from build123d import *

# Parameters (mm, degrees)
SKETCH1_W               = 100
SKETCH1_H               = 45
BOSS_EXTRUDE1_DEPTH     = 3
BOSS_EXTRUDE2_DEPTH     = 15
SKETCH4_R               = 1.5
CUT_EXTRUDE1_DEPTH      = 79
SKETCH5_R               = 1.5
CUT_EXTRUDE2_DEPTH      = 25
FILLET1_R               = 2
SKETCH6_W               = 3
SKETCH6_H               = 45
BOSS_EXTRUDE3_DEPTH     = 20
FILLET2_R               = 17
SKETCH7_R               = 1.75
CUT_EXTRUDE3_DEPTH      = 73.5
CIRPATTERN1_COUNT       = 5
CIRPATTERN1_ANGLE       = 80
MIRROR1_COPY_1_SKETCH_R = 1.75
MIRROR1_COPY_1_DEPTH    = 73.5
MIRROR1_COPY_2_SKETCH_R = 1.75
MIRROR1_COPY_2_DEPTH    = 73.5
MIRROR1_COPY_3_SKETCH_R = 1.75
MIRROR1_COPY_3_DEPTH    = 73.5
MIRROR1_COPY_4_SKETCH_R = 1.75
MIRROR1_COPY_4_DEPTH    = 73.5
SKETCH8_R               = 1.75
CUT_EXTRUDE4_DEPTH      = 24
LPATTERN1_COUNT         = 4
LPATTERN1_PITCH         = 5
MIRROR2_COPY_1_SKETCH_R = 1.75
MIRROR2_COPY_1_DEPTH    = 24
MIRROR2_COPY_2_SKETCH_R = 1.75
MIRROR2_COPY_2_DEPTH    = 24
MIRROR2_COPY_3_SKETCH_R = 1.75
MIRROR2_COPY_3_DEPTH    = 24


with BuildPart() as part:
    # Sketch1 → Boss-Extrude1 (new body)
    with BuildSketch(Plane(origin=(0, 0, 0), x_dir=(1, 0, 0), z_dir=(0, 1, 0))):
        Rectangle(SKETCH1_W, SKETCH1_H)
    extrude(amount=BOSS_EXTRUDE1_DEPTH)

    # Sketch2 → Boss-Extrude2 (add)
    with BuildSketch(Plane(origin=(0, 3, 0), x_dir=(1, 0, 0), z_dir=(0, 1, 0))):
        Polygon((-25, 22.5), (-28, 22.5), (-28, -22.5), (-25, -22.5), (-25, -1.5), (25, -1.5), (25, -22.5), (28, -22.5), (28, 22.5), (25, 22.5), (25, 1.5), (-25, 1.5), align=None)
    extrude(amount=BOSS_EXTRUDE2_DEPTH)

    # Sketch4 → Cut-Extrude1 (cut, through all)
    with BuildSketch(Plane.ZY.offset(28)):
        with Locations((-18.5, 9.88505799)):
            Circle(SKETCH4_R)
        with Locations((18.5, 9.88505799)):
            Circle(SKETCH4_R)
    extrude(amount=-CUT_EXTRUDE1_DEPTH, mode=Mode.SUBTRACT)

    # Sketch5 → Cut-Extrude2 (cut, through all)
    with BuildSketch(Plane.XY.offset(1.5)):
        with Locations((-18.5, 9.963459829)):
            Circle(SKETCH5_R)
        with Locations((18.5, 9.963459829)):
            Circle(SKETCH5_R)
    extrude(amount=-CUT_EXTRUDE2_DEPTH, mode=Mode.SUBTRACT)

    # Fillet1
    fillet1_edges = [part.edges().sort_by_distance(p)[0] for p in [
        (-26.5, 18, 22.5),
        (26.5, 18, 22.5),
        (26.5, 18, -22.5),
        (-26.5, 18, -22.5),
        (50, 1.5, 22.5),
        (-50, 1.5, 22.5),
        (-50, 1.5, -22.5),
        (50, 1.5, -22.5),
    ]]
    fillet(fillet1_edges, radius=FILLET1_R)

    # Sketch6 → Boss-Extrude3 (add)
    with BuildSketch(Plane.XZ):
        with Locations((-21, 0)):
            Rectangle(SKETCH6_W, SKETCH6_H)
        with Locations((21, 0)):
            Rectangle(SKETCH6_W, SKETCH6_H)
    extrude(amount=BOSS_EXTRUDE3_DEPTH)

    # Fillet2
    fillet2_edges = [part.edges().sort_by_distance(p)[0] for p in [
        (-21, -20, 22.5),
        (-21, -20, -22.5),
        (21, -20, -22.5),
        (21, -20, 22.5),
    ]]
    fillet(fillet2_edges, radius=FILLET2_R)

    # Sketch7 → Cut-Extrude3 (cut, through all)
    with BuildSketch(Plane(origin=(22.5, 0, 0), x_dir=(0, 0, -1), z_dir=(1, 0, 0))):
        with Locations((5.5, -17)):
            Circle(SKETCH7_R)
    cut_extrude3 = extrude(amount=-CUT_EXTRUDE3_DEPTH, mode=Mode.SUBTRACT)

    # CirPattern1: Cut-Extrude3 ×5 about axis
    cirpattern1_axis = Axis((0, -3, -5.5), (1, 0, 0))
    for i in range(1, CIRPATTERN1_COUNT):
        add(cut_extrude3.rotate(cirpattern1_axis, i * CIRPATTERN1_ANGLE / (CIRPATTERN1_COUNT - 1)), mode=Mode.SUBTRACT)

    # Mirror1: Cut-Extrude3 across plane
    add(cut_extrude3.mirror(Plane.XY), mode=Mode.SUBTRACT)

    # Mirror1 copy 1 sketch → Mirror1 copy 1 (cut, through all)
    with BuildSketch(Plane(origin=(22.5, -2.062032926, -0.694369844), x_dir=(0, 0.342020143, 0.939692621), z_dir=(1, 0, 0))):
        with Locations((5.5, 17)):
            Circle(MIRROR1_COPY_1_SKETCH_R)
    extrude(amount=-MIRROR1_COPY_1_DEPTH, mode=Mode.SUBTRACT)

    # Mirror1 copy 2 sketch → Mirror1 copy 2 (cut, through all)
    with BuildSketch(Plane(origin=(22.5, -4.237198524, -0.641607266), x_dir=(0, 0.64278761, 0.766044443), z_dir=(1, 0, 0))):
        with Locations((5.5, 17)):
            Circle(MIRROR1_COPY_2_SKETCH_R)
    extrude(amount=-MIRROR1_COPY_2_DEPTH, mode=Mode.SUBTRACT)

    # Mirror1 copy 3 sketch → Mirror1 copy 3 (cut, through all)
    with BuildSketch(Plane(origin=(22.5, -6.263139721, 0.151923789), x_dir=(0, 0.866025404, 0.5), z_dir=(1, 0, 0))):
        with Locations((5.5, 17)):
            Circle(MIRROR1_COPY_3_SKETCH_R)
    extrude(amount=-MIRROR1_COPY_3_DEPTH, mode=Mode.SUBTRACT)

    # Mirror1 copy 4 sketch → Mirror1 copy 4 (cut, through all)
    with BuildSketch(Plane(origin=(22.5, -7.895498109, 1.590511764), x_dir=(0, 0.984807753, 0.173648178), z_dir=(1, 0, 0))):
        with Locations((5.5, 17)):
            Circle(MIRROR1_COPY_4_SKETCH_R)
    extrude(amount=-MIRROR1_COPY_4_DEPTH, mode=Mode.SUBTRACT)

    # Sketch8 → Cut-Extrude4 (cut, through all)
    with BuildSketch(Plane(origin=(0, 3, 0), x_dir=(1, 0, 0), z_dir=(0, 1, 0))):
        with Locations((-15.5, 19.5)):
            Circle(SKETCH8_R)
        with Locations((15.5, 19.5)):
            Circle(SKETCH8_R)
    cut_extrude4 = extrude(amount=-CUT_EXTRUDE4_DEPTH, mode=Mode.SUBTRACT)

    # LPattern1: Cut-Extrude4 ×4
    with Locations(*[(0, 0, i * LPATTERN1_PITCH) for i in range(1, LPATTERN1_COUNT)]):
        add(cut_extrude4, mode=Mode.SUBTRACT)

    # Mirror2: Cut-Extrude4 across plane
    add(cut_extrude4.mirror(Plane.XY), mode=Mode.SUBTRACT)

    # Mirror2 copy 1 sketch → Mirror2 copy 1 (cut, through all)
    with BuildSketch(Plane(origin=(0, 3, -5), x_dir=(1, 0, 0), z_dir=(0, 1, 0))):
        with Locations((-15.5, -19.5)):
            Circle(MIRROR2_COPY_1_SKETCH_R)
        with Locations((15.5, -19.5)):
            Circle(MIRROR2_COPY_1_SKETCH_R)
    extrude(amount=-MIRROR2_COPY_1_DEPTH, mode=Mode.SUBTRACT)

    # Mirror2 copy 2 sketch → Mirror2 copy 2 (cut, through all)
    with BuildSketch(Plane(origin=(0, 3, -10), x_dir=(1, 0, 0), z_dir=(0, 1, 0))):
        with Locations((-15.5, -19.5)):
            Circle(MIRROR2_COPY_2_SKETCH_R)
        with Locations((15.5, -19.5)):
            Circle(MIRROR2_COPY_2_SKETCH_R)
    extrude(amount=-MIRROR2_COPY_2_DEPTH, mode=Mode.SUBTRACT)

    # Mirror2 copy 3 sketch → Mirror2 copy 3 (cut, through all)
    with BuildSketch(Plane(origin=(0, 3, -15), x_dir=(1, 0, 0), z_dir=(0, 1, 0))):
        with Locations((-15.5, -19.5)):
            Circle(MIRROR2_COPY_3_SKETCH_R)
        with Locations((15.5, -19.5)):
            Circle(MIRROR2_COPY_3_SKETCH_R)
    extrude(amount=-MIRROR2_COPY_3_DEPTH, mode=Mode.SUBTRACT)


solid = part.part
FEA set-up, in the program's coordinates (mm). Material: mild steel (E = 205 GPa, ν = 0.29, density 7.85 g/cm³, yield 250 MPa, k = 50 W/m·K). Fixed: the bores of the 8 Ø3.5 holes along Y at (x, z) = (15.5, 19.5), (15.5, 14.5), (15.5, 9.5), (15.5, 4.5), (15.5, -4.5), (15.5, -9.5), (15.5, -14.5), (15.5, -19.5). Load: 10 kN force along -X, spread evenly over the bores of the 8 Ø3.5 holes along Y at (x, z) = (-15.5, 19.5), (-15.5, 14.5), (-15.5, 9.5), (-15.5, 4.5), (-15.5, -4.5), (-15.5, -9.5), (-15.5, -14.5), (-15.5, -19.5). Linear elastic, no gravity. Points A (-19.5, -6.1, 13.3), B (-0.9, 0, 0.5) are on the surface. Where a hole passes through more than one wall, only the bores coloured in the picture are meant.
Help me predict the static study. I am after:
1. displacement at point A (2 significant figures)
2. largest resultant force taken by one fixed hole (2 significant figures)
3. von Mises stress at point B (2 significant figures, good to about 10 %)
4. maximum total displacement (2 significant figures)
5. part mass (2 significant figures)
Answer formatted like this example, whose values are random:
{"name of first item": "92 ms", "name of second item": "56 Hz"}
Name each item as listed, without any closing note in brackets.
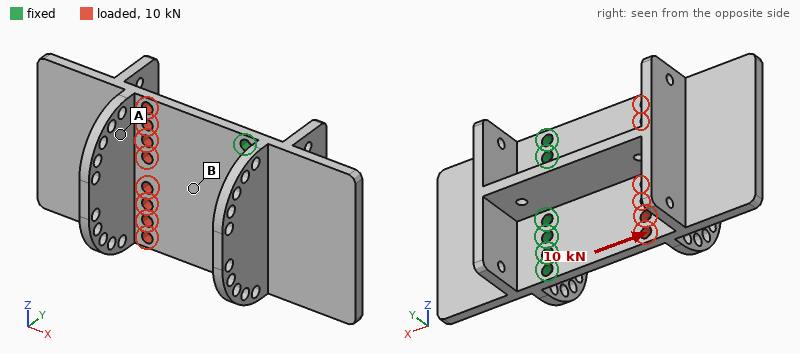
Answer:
{"displacement at point A": "21 µm", "largest resultant force taken by one fixed hole": "1.5 kN", "von Mises stress at point B": "71 MPa", "maximum total displacement": "40 µm", "part mass": "180 g"}
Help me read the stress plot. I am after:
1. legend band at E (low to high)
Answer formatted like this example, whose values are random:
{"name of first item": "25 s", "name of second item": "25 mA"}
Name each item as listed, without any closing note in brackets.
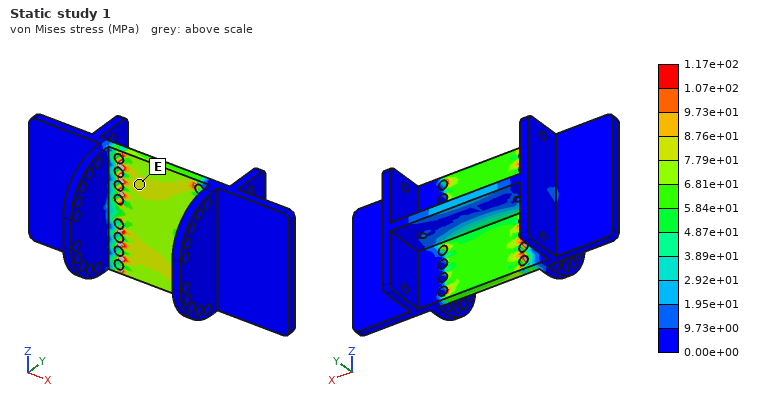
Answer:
{"legend band at E": "7.79e+01 to 8.76e+01 MPa"}
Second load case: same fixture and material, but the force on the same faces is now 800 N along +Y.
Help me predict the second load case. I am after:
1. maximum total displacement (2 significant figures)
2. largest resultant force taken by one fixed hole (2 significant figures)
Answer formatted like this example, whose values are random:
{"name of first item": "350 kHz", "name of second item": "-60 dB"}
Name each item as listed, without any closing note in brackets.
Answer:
{"maximum total displacement": "0.14 mm", "largest resultant force taken by one fixed hole": "710 N"}
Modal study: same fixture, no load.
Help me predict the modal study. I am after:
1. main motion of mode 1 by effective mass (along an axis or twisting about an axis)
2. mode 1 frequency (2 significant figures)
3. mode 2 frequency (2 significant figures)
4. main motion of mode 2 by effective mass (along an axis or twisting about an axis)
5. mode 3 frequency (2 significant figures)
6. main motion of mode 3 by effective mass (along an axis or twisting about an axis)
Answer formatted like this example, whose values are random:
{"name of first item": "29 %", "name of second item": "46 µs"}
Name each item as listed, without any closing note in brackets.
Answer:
{"main motion of mode 1 by effective mass": "along Y", "mode 1 frequency": "1300 Hz", "mode 2 frequency": "1700 Hz", "main motion of mode 2 by effective mass": "twisting about X", "mode 3 frequency": "3500 Hz", "main motion of mode 3 by effective mass": "along Y"}
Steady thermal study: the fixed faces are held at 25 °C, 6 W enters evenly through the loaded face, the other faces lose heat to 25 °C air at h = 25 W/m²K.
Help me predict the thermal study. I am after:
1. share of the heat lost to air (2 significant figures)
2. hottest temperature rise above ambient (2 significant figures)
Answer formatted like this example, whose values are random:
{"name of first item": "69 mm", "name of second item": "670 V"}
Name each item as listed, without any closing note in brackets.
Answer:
{"share of the heat lost to air": "43 %", "hottest temperature rise above ambient": "14 K"}
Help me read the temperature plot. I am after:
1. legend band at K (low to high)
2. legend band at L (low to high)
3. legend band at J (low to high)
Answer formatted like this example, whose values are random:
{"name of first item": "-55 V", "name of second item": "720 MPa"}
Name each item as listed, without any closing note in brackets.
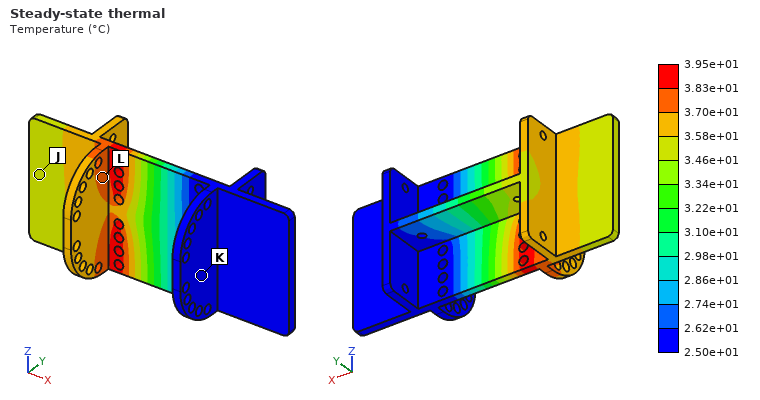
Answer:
{"legend band at K": "2.50e+01 to 2.62e+01 °C", "legend band at L": "3.70e+01 to 3.83e+01 °C", "legend band at J": "3.46e+01 to 3.58e+01 °C"}
